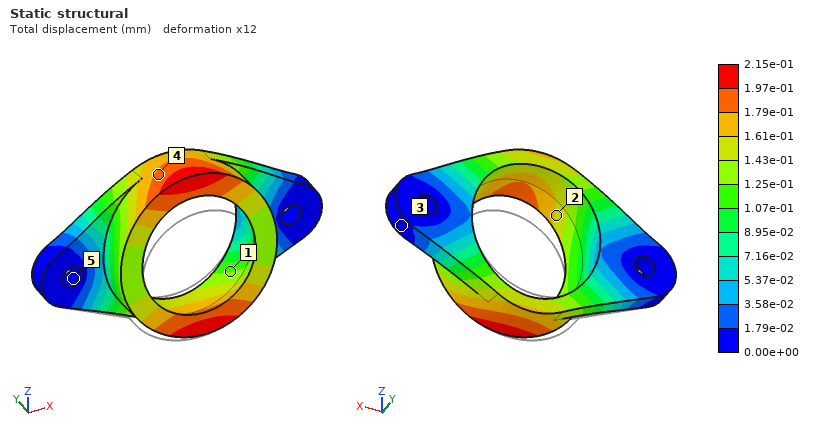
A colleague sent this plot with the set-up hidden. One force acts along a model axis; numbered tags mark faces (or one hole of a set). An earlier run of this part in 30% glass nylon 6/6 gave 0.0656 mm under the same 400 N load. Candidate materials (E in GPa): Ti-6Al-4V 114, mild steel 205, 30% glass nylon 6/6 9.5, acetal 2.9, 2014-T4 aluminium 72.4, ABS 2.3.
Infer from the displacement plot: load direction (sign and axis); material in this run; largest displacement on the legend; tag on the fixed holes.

+Z
acetal
2.15e-01 mm
5
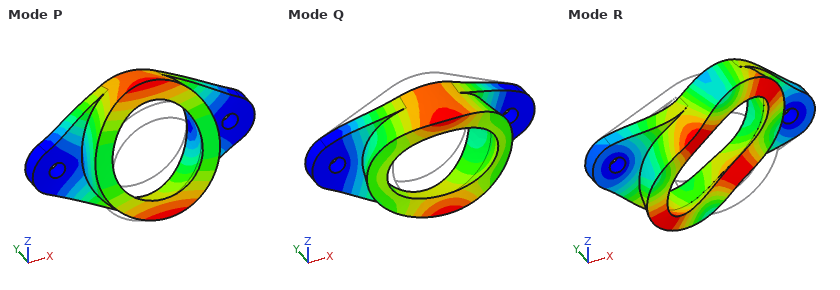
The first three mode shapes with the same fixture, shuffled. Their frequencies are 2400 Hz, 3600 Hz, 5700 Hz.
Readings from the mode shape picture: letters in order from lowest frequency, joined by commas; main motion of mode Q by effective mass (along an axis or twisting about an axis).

P, Q, R
along Y
